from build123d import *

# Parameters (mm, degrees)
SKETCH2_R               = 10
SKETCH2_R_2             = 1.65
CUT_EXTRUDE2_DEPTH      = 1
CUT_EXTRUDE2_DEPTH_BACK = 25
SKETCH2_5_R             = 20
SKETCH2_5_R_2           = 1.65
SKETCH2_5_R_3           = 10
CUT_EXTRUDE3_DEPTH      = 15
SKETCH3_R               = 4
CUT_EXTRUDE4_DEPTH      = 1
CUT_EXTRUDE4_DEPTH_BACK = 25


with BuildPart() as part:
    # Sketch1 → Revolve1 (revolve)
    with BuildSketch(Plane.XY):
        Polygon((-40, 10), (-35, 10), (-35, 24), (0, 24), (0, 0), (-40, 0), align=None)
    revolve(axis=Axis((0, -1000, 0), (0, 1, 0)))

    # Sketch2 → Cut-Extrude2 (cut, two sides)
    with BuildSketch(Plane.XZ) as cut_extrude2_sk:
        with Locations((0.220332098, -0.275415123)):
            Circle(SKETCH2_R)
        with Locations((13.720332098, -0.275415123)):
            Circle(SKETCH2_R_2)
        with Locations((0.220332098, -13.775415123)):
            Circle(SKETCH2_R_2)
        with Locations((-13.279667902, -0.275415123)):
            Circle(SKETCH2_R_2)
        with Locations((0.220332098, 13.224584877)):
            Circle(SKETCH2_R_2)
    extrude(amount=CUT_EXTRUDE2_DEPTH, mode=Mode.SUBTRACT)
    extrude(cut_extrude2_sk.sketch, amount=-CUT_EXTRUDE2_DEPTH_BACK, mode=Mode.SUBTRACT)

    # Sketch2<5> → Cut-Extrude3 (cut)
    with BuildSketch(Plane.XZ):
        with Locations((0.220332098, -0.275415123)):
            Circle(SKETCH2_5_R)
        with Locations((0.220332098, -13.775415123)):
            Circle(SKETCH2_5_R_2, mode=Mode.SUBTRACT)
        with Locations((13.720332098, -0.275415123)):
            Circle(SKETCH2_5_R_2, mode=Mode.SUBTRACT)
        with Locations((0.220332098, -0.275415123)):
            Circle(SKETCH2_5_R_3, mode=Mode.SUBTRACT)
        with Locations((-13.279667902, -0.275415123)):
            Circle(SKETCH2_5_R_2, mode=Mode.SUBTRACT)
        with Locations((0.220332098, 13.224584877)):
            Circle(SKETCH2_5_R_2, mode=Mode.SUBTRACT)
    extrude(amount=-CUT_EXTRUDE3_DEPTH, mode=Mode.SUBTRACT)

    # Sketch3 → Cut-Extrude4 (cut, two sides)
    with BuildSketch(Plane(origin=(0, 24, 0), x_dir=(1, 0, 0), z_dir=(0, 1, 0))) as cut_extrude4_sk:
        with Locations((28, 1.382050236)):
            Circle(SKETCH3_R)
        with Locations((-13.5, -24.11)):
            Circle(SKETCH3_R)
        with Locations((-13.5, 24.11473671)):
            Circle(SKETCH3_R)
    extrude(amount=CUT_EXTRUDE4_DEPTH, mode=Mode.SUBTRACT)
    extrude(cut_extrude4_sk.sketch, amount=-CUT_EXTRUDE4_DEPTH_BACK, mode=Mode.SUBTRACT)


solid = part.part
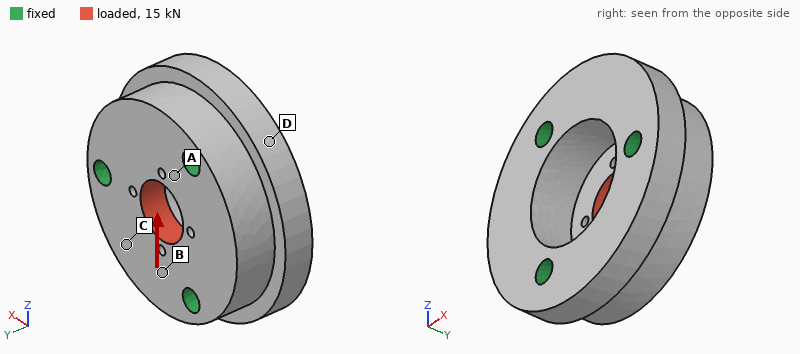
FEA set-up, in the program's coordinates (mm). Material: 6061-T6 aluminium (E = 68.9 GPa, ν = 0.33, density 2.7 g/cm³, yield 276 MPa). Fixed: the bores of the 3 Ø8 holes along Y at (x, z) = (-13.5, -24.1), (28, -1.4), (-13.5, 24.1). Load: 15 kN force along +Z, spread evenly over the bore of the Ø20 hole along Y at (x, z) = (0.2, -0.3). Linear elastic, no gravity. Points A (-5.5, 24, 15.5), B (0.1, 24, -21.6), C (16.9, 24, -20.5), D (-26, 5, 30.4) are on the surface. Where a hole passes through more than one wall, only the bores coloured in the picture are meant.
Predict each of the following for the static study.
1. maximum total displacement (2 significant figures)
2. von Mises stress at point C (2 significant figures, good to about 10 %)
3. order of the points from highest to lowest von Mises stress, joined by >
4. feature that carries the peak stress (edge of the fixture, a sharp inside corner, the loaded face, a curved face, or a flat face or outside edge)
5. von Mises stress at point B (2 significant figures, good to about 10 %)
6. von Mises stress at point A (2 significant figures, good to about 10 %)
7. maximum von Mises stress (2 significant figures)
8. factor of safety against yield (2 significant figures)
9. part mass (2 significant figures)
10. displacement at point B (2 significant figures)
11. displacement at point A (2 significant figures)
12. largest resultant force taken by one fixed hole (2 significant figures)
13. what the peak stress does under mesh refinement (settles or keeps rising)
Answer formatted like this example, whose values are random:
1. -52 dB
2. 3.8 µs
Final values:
1. 13 µm
2. 13 MPa
3. A > B > C > D
4. a curved face
5. 19 MPa
6. 34 MPa
7. 92 MPa
8. 3.0
9. 210 g
10. 6.6 µm
11. 5.6 µm
12. 5.2 kN
13. settles
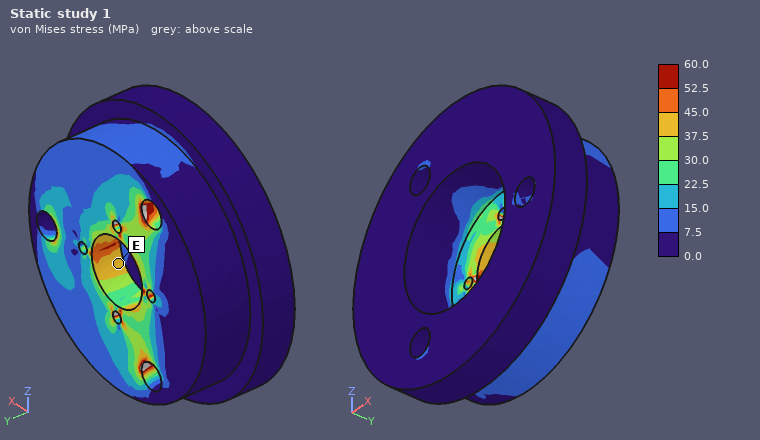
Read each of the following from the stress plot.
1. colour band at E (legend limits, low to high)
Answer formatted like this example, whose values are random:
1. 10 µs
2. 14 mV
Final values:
1. 37.5 to 45.0 MPa
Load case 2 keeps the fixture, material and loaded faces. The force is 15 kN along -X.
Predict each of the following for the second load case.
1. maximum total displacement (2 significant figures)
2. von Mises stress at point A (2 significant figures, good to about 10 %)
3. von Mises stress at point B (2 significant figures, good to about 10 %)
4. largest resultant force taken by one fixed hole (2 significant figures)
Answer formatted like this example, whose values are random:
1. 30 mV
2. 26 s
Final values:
1. 15 µm
2. 15 MPa
3. 10 MPa
4. 5.2 kN
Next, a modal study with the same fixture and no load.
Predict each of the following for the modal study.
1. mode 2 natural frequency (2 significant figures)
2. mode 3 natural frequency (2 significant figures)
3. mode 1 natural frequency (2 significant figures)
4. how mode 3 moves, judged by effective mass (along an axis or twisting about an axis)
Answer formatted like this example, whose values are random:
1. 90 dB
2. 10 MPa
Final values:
1. 18 kHz
2. 20 kHz
3. 18 kHz
4. along Y
